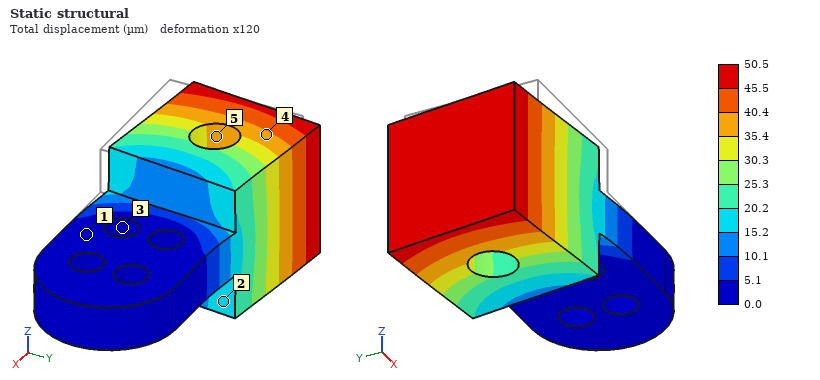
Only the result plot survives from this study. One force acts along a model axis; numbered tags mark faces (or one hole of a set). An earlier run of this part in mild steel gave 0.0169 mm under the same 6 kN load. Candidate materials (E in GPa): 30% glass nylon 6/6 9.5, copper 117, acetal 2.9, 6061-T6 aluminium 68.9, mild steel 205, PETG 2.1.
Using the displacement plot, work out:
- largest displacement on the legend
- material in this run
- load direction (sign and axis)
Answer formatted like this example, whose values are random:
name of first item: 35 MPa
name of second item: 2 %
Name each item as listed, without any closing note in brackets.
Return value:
largest displacement on the legend: 50.5 µm
material in this run: 6061-T6 aluminium
load direction: +Y
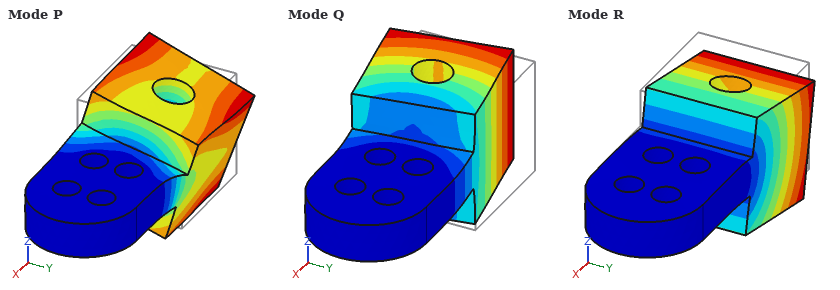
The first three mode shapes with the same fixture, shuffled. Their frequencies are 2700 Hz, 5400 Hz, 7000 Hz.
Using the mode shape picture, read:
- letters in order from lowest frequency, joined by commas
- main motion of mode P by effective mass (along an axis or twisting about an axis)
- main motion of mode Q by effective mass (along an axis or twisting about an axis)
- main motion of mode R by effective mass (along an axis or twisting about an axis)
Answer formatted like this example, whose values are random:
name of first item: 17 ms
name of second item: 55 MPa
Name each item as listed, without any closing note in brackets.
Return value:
letters in order from lowest frequency, joined by commas: R, Q, P
main motion of mode P by effective mass: twisting about X
main motion of mode Q by effective mass: along Y
main motion of mode R by effective mass: along Z
